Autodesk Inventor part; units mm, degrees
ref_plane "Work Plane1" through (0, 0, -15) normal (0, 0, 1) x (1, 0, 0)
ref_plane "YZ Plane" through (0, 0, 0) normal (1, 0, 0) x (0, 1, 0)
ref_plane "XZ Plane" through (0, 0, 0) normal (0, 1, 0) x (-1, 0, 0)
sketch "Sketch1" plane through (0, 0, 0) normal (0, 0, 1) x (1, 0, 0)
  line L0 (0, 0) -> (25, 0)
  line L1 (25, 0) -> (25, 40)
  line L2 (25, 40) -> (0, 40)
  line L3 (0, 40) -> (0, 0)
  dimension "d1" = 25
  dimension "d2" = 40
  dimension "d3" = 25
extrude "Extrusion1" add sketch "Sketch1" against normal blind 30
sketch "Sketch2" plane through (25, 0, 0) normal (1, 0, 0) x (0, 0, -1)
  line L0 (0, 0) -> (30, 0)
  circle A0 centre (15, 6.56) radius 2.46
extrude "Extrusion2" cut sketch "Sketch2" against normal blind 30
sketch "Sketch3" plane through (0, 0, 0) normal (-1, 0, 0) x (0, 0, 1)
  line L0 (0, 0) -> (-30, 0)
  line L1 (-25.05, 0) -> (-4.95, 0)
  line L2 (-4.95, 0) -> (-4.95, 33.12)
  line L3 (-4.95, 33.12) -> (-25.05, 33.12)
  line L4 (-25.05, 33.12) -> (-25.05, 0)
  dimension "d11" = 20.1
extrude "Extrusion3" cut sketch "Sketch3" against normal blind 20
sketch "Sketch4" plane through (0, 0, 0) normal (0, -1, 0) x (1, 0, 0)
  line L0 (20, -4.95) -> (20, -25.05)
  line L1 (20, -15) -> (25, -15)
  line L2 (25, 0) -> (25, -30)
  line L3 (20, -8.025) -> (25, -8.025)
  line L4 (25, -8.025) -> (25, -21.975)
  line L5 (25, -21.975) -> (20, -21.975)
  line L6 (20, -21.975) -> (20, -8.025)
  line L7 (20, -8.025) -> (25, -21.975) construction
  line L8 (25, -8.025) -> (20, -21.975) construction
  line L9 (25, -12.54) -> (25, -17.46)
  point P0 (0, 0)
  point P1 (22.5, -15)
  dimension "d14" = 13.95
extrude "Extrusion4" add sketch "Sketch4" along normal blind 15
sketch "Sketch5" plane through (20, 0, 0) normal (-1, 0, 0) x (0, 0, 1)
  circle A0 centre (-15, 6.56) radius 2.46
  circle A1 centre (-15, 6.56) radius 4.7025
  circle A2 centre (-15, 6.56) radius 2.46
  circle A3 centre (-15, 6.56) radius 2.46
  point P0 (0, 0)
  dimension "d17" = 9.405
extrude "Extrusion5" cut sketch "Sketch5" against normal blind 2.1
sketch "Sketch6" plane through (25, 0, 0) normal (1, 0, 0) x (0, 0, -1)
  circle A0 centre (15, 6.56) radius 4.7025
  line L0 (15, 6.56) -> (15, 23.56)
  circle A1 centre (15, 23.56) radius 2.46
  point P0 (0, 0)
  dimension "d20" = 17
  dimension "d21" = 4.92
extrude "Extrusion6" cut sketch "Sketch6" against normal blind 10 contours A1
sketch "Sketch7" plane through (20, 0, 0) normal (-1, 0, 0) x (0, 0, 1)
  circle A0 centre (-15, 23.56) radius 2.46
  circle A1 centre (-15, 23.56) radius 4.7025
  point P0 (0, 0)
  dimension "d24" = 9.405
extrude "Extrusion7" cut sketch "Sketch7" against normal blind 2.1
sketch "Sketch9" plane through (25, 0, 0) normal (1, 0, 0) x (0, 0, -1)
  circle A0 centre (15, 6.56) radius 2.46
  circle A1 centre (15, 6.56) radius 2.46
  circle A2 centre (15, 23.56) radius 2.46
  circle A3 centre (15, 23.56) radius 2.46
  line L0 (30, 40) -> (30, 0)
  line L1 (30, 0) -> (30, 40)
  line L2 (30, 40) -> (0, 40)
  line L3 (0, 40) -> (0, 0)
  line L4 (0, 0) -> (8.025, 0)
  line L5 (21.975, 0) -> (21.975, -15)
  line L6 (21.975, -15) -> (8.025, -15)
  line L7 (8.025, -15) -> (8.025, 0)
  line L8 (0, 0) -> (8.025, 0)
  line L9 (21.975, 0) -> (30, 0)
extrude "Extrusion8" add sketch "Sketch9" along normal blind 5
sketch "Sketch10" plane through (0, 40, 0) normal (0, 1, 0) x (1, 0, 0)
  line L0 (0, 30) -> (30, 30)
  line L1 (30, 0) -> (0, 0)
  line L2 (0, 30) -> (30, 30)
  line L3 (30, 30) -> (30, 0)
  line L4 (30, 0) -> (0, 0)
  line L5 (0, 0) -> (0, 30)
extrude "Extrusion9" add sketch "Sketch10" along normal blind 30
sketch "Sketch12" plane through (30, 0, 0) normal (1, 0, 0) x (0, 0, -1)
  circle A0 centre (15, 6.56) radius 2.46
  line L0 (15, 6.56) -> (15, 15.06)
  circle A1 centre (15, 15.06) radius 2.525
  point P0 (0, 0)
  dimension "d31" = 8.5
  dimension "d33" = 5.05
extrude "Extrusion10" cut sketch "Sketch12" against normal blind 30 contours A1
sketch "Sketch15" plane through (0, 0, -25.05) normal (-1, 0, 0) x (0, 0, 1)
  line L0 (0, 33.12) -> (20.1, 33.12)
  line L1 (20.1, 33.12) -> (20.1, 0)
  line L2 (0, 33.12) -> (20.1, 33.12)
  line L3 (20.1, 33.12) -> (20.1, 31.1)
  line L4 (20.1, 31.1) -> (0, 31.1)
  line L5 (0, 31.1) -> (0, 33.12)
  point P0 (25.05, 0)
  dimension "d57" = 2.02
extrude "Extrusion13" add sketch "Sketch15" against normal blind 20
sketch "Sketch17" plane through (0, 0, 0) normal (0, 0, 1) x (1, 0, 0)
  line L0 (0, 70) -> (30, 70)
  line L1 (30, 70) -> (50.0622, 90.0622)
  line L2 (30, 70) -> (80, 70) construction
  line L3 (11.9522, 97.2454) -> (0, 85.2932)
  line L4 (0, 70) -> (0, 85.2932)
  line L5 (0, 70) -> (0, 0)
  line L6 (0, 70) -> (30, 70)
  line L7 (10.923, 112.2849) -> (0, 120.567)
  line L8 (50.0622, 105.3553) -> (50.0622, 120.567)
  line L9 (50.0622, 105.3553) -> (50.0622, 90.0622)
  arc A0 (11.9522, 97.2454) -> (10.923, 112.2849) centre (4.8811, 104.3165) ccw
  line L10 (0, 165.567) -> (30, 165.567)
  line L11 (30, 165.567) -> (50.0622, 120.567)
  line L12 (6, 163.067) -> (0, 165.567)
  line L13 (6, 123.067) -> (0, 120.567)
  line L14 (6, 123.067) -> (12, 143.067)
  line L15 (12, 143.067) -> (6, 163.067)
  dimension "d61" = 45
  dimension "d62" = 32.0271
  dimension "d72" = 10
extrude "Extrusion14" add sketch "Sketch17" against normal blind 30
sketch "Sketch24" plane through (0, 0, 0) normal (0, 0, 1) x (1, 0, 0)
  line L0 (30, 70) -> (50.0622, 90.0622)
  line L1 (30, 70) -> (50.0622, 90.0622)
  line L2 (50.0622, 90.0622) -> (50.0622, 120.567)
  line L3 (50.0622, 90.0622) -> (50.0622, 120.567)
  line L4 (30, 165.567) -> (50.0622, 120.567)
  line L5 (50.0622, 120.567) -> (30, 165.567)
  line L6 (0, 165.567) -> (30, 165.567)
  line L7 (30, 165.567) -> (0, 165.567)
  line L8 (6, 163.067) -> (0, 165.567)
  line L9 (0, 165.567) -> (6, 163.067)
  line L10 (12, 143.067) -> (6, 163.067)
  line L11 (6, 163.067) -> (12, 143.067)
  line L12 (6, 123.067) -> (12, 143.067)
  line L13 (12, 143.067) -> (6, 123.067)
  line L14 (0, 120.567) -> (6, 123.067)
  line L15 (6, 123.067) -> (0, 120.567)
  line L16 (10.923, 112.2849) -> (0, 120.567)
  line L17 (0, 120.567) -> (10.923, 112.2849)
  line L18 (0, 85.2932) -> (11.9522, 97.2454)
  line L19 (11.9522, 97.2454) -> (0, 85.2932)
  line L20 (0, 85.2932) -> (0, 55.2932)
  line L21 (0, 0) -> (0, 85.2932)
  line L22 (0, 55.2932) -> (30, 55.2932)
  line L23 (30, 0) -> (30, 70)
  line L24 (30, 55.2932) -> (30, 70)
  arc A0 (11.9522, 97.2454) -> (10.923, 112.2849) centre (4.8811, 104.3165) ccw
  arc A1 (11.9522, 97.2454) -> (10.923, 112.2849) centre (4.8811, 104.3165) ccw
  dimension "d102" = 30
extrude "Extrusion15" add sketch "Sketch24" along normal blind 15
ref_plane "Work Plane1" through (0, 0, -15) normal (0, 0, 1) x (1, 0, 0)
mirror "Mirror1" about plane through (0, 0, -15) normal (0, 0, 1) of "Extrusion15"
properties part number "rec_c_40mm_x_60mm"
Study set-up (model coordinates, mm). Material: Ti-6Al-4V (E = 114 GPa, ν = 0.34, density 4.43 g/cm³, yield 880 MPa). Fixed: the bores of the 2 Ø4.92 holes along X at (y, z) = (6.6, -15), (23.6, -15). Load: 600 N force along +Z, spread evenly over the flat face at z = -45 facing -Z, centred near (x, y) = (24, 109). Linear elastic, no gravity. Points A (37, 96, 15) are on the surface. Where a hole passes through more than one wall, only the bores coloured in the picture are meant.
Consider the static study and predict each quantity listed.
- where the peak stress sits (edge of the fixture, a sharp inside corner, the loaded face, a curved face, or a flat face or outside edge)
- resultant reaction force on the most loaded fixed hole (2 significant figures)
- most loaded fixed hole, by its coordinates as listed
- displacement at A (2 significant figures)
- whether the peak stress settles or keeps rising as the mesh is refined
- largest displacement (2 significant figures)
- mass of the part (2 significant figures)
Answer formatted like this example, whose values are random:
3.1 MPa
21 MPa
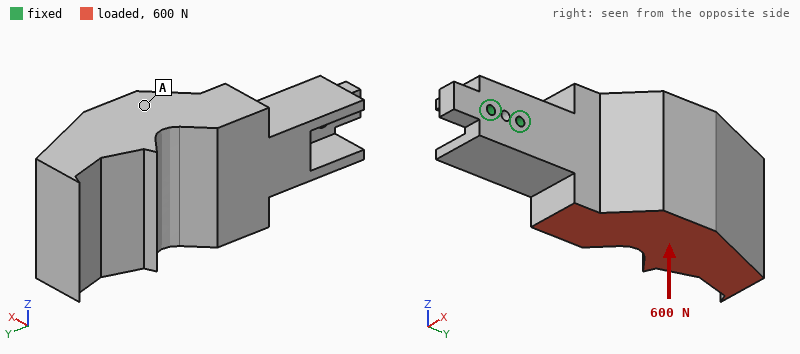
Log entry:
edge of the fixture
2.8 kN
(23.6, -15)
51 µm
keeps rising
93 µm
1.2 kg
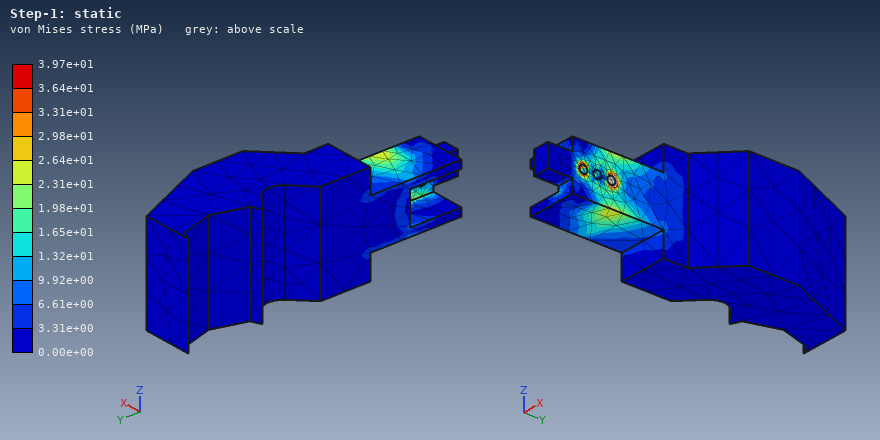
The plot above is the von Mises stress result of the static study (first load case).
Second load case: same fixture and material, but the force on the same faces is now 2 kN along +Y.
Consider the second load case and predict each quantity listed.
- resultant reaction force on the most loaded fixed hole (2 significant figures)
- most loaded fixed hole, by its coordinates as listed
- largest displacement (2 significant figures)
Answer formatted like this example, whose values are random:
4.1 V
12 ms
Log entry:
3.0 kN
(23.6, -15)
0.12 mm
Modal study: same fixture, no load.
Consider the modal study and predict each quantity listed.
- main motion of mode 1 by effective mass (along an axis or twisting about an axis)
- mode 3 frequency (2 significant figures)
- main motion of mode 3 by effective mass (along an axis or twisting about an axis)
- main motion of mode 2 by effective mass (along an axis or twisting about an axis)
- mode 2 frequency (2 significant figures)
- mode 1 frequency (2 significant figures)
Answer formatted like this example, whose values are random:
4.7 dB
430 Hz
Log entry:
along X
1200 Hz
twisting about Y
along Z
480 Hz
420 Hz
